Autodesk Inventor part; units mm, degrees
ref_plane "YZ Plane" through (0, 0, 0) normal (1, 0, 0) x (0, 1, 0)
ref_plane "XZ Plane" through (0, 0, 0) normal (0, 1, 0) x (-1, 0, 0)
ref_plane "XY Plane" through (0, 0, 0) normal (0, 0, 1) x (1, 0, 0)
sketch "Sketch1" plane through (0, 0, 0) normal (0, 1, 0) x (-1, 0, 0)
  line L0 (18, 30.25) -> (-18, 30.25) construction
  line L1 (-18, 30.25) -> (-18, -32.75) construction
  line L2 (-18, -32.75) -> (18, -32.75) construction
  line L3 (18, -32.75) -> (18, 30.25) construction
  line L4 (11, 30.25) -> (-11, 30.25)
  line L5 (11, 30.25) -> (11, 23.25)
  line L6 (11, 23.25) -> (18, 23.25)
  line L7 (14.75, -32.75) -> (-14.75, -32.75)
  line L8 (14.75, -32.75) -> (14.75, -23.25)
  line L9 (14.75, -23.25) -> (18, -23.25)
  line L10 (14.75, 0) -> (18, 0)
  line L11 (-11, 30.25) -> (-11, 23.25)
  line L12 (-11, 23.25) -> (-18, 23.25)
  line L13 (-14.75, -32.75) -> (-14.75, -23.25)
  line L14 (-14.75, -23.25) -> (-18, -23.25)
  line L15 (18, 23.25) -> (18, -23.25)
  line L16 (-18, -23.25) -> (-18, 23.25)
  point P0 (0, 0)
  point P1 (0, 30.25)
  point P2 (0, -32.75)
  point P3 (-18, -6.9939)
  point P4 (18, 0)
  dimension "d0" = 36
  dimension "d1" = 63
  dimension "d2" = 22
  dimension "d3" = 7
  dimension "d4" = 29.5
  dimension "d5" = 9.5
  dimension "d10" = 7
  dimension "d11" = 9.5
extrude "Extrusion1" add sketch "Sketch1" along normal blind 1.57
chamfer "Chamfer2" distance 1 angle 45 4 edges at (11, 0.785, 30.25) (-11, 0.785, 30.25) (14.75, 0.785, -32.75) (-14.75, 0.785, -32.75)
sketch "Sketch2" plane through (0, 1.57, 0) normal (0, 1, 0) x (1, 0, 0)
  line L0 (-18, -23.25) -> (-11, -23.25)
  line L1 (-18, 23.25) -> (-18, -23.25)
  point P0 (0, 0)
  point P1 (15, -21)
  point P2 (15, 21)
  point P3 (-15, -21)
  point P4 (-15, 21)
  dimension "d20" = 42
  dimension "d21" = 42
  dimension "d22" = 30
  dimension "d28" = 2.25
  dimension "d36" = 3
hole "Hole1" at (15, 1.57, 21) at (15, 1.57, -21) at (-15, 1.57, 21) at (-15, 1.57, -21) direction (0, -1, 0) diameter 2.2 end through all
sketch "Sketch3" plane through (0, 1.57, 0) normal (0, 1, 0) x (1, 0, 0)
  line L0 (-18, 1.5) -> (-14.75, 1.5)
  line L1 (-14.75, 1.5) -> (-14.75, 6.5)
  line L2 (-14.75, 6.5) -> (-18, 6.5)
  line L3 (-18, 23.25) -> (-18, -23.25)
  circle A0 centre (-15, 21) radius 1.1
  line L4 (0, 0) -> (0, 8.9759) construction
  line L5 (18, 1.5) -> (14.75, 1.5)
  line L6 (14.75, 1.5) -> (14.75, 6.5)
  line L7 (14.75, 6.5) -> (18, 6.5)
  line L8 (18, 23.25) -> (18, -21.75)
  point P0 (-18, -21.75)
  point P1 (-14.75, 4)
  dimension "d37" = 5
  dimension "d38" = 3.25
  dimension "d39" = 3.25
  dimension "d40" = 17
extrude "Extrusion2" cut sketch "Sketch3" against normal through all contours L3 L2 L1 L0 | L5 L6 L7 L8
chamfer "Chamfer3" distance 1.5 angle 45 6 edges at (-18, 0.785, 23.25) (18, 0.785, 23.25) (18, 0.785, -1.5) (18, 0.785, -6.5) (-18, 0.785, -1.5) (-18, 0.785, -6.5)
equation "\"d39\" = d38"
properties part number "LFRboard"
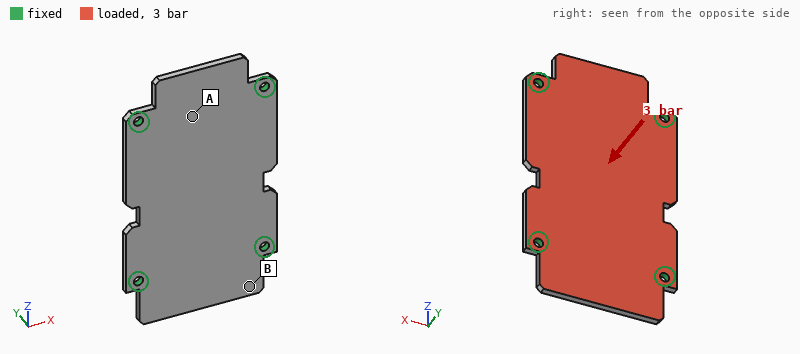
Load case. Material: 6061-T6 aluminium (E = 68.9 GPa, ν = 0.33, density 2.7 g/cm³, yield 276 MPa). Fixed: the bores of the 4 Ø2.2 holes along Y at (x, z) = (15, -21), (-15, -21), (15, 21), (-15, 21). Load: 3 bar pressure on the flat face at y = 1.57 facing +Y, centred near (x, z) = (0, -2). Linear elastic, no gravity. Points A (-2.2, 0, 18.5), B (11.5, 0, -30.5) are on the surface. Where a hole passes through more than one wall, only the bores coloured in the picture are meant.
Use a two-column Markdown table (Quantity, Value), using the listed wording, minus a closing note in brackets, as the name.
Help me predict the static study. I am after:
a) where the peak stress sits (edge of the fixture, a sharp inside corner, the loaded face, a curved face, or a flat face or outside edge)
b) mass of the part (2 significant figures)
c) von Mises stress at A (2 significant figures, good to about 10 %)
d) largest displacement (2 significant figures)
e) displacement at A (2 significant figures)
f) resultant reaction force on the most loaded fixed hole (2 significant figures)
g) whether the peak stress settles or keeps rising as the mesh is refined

| Quantity | Value |
|---|---|
| where the peak stress sits | edge of the fixture |
| mass of the part | 8.7 g |
| von Mises stress at A | 44 MPa |
| largest displacement | 0.16 mm |
| displacement at A | 0.063 mm |
| resultant reaction force on the most loaded fixed hole | 160 N |
| whether the peak stress settles or keeps rising as the mesh is refined | keeps rising |
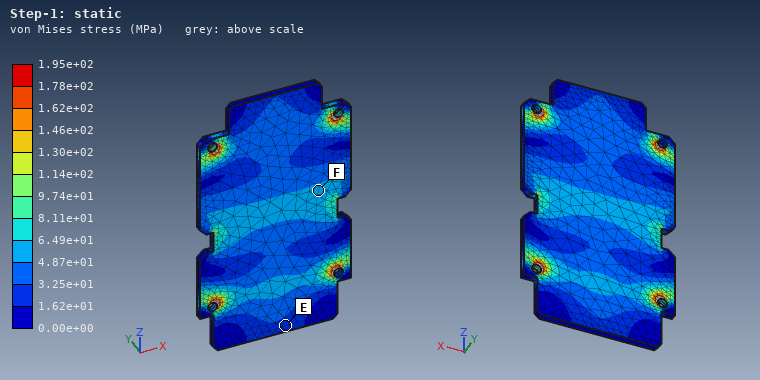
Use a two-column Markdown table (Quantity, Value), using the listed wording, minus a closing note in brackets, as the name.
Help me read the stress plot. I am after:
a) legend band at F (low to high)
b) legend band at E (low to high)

| Quantity | Value |
|---|---|
| legend band at F | 4.87e+01 to 6.49e+01 MPa |
| legend band at E | 1.62e+01 to 3.25e+01 MPa |
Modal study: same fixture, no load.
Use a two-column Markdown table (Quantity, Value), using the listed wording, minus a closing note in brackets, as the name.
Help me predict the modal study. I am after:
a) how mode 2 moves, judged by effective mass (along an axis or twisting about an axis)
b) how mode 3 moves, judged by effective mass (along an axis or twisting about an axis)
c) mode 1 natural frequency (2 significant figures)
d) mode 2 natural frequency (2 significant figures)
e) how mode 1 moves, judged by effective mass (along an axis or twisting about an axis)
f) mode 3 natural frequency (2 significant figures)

| Quantity | Value |
|---|---|
| how mode 2 moves, judged by effective mass | along Y |
| how mode 3 moves, judged by effective mass | twisting about Z |
| mode 1 natural frequency | 3700 Hz |
| mode 2 natural frequency | 5700 Hz |
| how mode 1 moves, judged by effective mass | along Y |
| mode 3 natural frequency | 6100 Hz |
